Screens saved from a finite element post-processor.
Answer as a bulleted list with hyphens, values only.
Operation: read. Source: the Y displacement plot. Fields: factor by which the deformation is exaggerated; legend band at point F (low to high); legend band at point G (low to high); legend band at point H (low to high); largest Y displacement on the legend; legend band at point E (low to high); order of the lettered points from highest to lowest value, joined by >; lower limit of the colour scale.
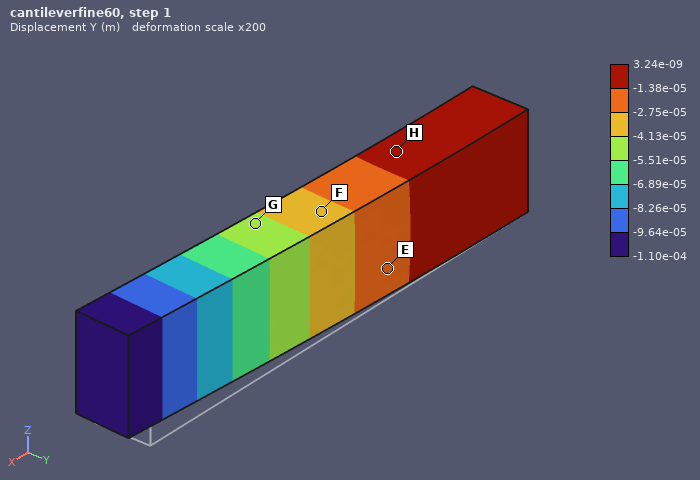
- 200
- -4.13e-05 to -2.75e-05 m
- -5.51e-05 to -4.13e-05 m
- -1.38e-05 to 3.24e-09 m
- 3.24e-09 m
- -2.75e-05 to -1.38e-05 m
- H > E > F > G
- -1.10e-04 m
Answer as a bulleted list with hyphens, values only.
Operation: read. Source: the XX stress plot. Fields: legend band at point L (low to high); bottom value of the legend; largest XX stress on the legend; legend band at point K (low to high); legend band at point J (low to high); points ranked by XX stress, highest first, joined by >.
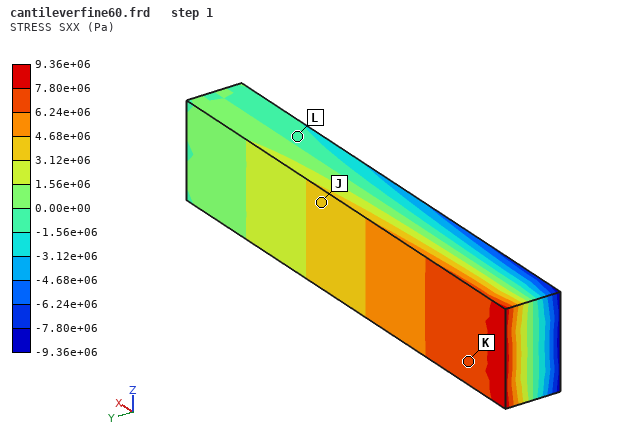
- -1.56e+06 to 0.00e+00 Pa
- -9.36e+06 Pa
- 9.36e+06 Pa
- 6.24e+06 to 7.80e+06 Pa
- 3.12e+06 to 4.68e+06 Pa
- K > J > L
